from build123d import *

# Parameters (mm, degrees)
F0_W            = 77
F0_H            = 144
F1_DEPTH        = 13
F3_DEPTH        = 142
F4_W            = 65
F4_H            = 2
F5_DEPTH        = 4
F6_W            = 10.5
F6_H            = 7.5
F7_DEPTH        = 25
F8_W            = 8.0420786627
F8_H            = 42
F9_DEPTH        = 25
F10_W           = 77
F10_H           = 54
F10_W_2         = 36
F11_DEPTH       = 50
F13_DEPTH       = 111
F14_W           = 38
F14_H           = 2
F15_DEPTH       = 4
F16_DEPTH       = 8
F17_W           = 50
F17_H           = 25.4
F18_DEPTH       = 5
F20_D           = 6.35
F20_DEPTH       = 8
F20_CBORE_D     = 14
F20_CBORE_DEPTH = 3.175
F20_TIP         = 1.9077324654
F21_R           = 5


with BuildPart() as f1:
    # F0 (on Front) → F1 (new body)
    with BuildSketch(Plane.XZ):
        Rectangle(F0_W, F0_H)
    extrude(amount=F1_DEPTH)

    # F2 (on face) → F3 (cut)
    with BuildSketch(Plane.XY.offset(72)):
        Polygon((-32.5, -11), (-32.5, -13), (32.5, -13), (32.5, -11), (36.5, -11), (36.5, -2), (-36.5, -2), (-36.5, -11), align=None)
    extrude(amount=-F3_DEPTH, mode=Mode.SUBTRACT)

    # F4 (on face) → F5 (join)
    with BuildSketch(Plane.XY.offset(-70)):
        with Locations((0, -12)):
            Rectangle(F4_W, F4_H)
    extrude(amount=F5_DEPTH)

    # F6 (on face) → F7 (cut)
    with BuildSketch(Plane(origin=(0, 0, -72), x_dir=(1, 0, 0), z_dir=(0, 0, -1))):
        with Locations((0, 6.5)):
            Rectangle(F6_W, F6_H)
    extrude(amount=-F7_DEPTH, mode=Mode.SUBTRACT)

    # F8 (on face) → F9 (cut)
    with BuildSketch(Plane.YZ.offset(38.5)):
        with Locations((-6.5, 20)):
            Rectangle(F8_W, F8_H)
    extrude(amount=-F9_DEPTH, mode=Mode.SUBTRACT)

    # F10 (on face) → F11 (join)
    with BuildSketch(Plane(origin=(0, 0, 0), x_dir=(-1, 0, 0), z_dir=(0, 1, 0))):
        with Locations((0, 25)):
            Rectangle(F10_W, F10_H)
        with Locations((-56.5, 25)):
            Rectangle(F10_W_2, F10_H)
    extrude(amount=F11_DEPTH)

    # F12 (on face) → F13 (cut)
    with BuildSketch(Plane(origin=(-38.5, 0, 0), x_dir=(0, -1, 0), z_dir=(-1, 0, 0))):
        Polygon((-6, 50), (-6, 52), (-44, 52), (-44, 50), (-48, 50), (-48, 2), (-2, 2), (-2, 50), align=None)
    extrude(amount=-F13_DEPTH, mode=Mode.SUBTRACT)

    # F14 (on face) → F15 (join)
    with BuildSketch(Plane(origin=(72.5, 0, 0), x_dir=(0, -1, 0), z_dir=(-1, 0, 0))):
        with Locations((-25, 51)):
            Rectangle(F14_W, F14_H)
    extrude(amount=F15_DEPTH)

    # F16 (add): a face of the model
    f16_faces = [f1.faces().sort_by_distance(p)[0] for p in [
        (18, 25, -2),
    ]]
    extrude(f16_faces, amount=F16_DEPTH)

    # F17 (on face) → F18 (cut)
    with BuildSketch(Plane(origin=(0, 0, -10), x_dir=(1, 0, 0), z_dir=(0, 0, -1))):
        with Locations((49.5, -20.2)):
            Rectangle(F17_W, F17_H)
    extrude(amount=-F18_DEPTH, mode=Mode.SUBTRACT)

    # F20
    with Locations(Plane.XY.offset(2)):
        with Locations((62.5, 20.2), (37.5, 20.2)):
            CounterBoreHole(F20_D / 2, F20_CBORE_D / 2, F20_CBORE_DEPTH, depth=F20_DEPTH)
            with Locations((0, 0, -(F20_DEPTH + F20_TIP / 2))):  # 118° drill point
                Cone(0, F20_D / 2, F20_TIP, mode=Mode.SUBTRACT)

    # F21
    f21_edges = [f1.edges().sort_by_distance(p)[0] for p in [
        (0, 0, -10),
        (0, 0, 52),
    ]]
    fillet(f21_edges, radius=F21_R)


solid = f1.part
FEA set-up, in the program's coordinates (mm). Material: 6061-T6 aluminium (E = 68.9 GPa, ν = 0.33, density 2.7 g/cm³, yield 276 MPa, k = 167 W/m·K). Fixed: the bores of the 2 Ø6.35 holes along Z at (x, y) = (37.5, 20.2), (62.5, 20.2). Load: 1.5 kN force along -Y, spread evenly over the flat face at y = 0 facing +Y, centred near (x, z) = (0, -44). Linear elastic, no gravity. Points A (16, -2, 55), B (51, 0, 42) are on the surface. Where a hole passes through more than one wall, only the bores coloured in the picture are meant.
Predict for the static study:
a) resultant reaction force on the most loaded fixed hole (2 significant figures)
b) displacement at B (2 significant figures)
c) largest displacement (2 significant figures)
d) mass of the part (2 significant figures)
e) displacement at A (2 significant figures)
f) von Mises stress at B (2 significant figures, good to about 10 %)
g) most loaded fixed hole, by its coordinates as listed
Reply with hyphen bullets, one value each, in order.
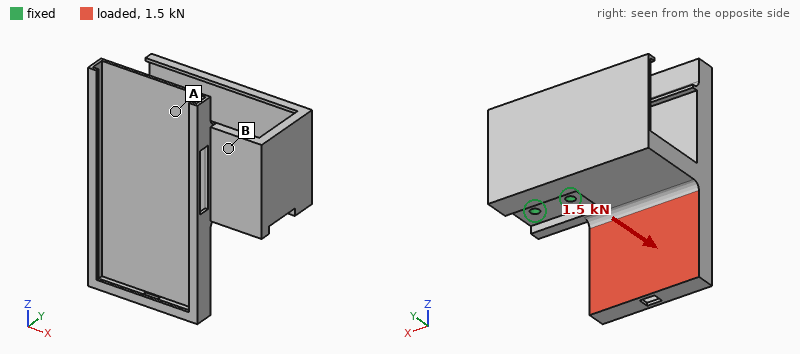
- 3.4 kN
- 0.35 mm
- 1.5 mm
- 330 g
- 0.67 mm
- 28 MPa
- (37.5, 20.2)
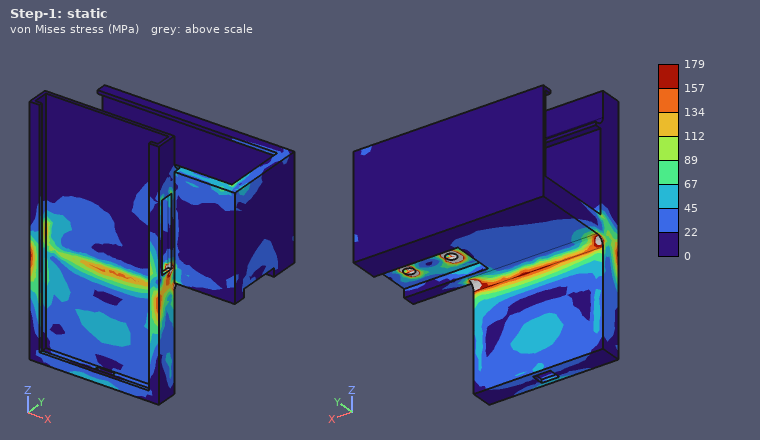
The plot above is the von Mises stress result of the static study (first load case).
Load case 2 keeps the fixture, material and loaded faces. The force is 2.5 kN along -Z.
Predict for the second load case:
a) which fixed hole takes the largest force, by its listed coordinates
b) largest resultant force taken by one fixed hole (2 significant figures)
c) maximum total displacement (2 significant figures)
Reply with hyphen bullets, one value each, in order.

- (37.5, 20.2)
- 5.3 kN
- 0.90 mm
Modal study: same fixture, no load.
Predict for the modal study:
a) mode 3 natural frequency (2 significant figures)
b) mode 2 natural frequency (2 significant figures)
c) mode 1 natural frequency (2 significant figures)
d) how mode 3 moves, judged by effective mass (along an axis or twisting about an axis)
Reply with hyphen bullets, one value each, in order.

- 950 Hz
- 770 Hz
- 590 Hz
- along Z
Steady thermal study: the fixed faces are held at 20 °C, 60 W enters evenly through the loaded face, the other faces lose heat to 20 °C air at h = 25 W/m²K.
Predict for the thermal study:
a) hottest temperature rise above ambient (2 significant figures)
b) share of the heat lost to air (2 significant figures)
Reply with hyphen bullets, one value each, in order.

- 63 K
- 44 %
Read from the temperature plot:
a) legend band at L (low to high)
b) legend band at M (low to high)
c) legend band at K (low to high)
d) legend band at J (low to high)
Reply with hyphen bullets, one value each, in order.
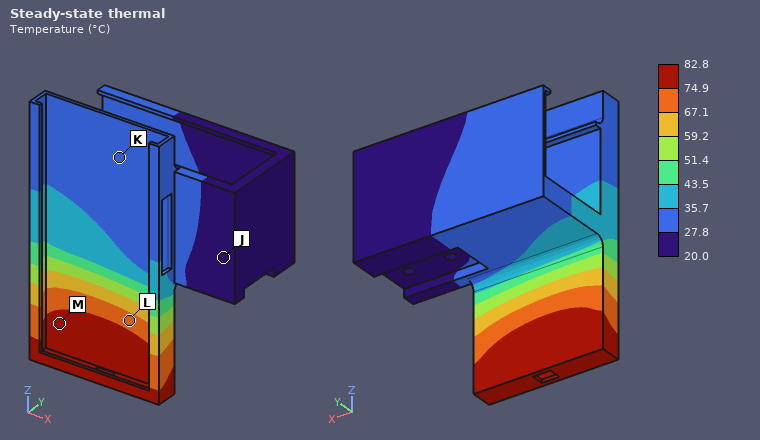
- 67.1 to 74.9 °C
- 74.9 to 82.8 °C
- 27.8 to 35.7 °C
- 20.0 to 27.8 °C
